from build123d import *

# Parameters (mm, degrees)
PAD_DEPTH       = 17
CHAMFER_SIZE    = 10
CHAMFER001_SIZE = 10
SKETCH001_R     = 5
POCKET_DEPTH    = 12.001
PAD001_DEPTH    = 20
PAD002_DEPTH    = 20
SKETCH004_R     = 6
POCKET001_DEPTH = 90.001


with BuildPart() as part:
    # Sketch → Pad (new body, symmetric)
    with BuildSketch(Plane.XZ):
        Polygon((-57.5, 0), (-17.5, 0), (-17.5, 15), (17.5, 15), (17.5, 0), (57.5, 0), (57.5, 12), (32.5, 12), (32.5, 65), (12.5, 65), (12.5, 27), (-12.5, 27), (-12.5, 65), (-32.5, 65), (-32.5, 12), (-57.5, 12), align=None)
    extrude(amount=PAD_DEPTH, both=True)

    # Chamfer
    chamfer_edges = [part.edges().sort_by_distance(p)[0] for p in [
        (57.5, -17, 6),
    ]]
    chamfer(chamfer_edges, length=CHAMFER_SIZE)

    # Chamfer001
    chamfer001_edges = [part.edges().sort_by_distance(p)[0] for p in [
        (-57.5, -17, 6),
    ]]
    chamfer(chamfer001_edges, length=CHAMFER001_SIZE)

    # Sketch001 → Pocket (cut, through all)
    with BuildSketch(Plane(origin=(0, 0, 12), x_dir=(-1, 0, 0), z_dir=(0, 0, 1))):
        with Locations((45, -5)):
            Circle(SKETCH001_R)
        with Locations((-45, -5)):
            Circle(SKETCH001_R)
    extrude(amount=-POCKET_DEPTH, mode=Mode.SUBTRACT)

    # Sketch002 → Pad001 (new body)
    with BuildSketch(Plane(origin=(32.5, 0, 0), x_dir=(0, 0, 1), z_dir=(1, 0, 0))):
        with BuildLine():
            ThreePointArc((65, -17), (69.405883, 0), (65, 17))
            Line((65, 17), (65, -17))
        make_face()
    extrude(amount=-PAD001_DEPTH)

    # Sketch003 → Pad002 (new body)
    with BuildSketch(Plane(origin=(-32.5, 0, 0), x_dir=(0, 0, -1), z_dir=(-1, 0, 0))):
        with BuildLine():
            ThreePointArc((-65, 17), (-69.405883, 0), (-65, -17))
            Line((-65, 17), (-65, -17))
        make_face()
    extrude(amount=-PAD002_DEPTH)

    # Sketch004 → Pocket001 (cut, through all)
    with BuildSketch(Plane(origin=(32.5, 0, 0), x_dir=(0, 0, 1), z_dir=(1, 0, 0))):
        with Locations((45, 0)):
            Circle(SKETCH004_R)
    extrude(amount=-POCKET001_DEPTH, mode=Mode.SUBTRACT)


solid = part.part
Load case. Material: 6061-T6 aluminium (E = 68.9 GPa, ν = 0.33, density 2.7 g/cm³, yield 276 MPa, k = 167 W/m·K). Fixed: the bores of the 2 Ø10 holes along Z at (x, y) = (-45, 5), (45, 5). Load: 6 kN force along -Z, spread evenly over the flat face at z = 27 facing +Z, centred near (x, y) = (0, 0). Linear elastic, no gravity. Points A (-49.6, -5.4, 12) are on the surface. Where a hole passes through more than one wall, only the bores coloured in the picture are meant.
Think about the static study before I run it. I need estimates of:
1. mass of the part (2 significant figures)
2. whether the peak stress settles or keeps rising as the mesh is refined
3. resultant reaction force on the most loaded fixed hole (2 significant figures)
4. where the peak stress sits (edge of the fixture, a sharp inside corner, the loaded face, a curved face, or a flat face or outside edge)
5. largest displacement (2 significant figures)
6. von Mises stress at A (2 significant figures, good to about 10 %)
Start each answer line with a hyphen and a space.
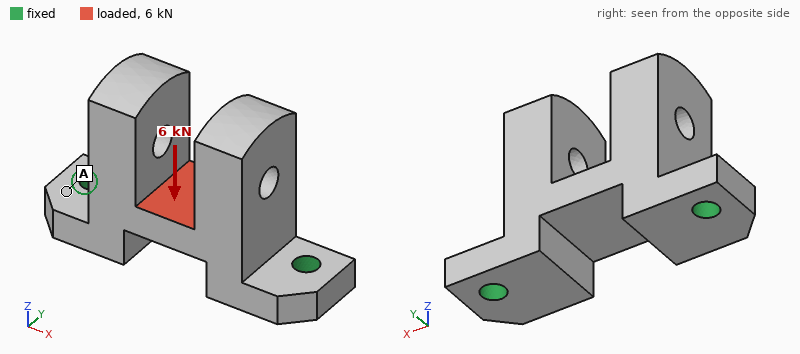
- 300 g
- keeps rising
- 4.9 kN
- edge of the fixture
- 50 µm
- 7.3 MPa
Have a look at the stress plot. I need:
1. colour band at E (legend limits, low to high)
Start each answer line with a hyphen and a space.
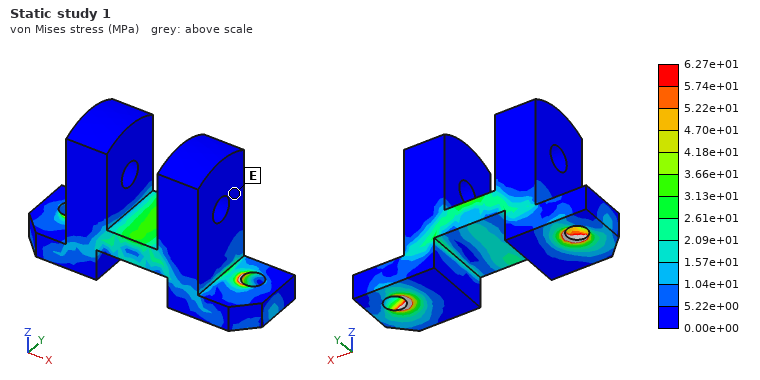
- 0.00e+00 to 5.22e+00 MPa
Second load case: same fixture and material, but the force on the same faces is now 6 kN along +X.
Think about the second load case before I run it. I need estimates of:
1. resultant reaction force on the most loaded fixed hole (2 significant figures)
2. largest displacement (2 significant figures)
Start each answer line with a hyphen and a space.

- 3.4 kN
- 16 µm
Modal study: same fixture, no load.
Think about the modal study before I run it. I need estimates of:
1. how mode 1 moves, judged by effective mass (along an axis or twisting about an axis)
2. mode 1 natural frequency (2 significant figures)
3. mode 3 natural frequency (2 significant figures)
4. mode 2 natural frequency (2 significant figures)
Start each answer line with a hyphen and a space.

- along Y
- 2000 Hz
- 4200 Hz
- 3500 Hz
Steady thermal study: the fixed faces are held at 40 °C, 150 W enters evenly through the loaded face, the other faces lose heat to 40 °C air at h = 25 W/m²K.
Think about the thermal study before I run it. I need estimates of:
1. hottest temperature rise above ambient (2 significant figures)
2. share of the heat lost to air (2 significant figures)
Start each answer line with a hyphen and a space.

- 44 K
- 8.3 %
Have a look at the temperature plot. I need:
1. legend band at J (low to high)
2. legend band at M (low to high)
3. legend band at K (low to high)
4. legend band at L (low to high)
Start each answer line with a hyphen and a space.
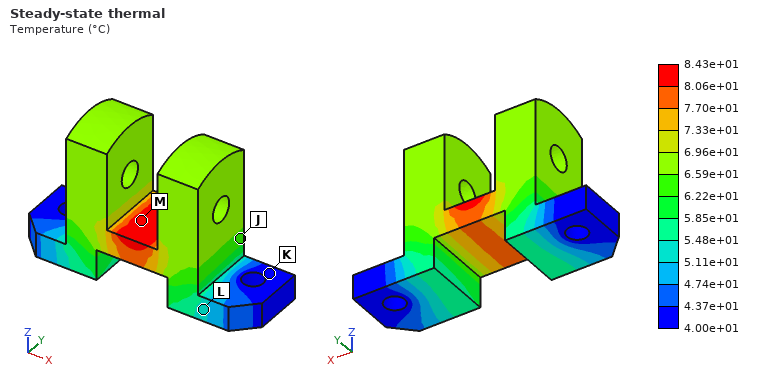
- 6.22e+01 to 6.59e+01 °C
- 8.06e+01 to 8.43e+01 °C
- 4.00e+01 to 4.37e+01 °C
- 5.11e+01 to 5.48e+01 °C
